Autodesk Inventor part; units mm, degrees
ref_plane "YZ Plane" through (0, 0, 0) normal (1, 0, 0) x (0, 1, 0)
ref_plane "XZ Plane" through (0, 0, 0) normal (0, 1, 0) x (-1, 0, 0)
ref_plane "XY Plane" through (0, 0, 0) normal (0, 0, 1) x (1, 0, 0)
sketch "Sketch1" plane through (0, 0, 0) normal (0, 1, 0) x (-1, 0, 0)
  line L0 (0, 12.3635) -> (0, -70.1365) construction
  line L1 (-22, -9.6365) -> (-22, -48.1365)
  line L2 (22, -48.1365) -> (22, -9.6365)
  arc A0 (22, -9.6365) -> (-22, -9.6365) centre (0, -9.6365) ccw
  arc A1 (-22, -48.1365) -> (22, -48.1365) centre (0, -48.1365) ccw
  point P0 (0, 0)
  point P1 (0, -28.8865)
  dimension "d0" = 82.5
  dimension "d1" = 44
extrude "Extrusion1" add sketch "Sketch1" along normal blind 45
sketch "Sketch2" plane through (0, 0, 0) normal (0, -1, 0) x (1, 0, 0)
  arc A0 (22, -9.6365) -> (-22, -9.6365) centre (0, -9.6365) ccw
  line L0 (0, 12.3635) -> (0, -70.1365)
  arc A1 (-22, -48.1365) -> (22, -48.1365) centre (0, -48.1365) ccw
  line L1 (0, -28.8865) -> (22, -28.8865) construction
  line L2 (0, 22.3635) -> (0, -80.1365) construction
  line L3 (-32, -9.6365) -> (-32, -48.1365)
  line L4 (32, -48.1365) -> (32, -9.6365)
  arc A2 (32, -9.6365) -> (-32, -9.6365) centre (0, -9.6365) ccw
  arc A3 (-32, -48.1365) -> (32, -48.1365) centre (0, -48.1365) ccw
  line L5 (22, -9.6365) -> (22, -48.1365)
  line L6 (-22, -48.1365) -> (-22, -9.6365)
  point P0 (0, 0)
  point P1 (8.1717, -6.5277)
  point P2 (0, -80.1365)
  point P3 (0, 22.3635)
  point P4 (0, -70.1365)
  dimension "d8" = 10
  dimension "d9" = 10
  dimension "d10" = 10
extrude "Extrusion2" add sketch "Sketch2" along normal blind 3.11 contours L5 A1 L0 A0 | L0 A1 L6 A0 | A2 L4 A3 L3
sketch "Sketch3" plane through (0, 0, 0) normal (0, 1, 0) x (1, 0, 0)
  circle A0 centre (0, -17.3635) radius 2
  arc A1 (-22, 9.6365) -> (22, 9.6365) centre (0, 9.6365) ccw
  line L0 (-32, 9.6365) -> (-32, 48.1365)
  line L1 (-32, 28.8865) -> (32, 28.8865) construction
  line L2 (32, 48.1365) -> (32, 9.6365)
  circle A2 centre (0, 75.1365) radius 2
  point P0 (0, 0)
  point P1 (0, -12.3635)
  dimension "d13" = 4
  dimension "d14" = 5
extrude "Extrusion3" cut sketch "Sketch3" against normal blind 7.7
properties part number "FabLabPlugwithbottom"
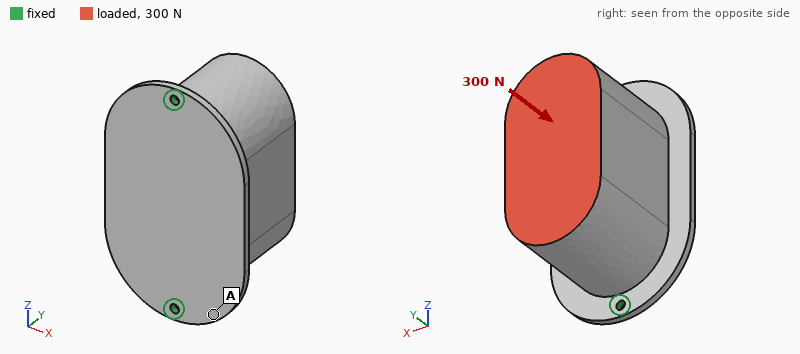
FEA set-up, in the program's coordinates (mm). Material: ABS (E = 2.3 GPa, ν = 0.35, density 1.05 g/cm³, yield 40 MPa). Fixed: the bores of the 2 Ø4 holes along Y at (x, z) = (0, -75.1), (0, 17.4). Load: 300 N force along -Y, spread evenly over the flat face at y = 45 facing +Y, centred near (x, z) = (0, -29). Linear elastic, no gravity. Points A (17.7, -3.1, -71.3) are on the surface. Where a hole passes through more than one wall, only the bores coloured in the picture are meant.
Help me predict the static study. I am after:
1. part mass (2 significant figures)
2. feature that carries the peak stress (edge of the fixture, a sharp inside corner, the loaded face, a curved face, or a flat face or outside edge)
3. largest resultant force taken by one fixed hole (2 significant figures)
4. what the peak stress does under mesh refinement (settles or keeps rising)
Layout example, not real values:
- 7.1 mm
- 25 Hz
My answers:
- 170 g
- edge of the fixture
- 170 N
- keeps rising
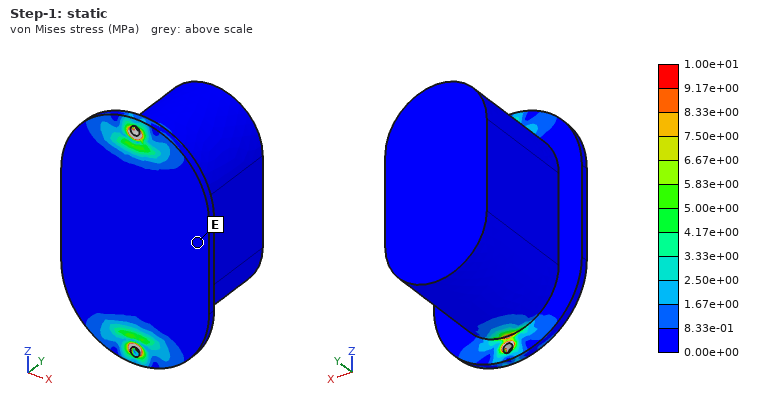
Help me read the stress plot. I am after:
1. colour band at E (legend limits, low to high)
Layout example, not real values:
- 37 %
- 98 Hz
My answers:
- 0.00e+00 to 8.33e-01 MPa
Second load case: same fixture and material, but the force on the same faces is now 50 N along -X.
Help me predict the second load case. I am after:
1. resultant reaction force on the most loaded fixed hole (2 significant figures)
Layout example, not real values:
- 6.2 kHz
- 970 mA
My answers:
- 25 N
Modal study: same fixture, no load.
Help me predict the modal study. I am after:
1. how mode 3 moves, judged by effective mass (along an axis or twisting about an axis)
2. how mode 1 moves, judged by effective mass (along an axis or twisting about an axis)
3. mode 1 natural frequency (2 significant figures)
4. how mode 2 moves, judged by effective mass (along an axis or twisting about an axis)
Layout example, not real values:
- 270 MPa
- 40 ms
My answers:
- along Z
- along X
- 120 Hz
- along Y
